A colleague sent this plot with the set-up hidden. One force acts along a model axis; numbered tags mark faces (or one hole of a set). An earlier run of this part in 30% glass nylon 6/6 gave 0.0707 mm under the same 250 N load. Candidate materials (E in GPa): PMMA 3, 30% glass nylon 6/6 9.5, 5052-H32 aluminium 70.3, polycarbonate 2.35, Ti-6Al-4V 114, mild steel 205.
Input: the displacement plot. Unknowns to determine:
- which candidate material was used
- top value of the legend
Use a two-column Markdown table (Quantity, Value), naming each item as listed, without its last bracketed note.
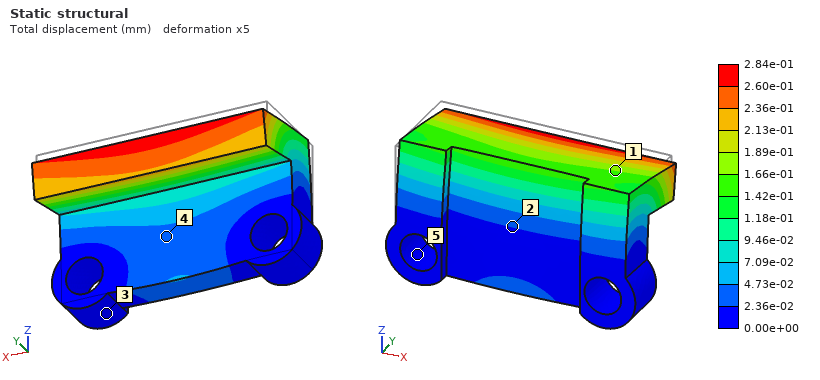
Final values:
| Quantity | Value |
|---|---|
| which candidate material was used | polycarbonate |
| top value of the legend | 2.84e-01 mm |
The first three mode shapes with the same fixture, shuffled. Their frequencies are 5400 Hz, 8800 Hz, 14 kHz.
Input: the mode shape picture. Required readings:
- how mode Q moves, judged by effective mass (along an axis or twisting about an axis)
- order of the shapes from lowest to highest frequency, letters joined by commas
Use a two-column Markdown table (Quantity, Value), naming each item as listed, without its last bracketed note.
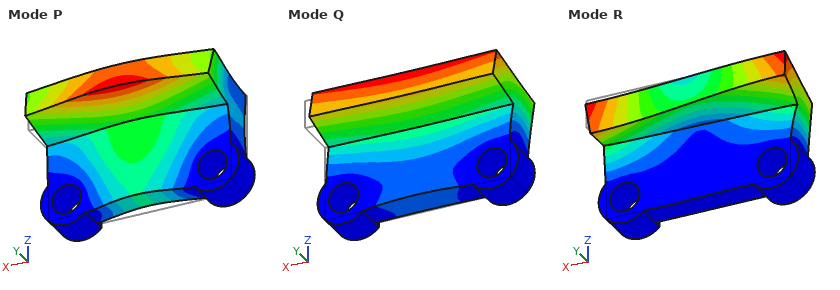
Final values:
| Quantity | Value |
|---|---|
| how mode Q moves, judged by effective mass | along Y |
| order of the shapes from lowest to highest frequency, letters joined by commas | Q, R, P |
